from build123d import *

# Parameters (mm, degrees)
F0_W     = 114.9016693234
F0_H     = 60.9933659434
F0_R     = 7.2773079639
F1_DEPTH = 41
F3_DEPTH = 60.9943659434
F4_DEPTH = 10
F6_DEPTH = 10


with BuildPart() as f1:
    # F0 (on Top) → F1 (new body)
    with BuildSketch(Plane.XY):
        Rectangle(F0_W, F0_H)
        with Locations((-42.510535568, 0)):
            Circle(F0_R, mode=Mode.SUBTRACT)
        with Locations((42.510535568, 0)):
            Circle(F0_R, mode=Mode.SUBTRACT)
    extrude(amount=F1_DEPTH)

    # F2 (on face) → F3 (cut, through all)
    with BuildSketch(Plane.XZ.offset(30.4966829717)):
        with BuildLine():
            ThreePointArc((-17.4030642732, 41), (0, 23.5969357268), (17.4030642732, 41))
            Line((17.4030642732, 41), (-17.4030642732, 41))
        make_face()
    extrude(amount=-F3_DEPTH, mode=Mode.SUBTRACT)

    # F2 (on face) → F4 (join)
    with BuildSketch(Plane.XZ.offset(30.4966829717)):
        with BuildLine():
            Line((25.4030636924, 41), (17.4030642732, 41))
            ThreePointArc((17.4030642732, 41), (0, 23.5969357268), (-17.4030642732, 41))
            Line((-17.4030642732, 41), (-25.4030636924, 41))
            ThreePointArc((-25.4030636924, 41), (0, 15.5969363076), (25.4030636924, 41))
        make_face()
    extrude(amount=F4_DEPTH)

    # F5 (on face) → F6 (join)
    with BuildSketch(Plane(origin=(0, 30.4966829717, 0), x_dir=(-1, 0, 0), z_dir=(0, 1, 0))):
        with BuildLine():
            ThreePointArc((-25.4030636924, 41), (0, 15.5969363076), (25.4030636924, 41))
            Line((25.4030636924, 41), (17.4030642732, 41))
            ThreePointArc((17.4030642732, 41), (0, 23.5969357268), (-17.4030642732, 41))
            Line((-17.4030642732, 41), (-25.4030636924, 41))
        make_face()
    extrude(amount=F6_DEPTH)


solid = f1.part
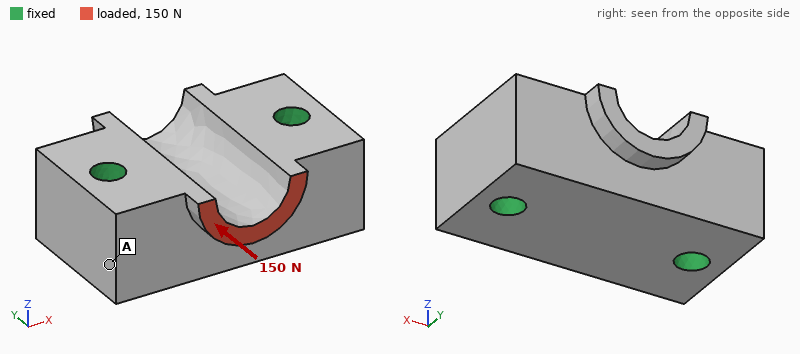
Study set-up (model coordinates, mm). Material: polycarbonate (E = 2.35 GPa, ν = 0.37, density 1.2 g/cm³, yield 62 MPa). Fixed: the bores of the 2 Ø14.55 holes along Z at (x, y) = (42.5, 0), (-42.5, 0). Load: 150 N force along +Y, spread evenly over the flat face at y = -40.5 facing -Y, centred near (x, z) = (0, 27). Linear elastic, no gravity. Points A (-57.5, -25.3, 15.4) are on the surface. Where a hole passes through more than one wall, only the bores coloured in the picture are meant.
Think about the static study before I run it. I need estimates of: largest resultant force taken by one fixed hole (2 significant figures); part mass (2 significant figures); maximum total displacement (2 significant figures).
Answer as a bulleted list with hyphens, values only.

- 78 N
- 310 g
- 6.2 µm
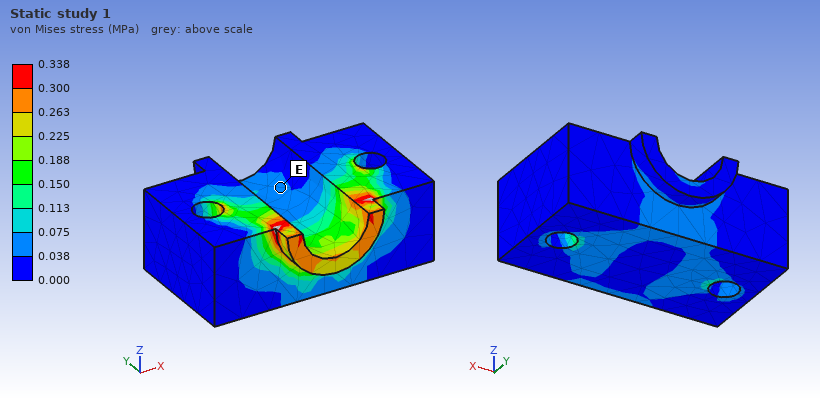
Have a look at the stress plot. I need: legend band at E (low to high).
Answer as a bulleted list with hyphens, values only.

- 0.038 to 0.075 MPa
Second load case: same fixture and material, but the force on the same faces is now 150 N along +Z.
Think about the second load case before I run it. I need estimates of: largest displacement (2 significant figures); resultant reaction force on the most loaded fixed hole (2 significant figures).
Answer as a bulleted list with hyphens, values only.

- 24 µm
- 78 N
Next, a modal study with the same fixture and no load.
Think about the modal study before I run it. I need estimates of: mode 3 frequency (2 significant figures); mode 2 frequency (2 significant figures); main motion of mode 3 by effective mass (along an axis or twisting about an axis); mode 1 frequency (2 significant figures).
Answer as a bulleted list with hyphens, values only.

- 4200 Hz
- 3700 Hz
- along Y
- 3600 Hz
